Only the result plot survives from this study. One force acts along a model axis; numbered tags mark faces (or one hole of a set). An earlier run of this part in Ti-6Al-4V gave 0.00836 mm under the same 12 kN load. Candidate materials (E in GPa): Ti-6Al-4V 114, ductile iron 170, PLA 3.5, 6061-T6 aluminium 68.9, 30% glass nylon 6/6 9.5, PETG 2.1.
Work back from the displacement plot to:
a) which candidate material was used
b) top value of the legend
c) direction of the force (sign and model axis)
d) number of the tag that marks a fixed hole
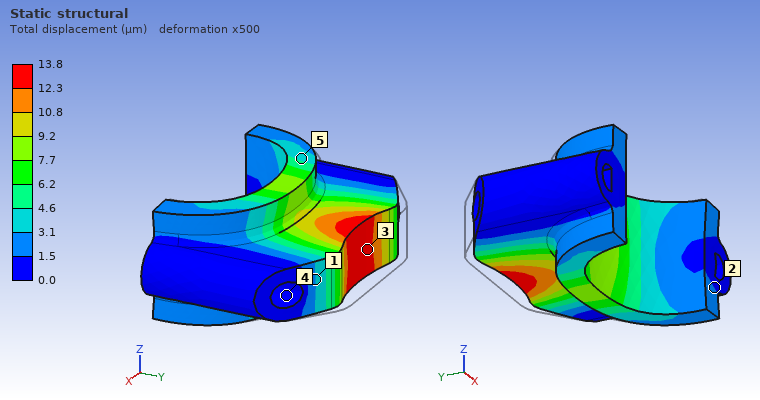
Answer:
6061-T6 aluminium
13.8 µm
-Y
4
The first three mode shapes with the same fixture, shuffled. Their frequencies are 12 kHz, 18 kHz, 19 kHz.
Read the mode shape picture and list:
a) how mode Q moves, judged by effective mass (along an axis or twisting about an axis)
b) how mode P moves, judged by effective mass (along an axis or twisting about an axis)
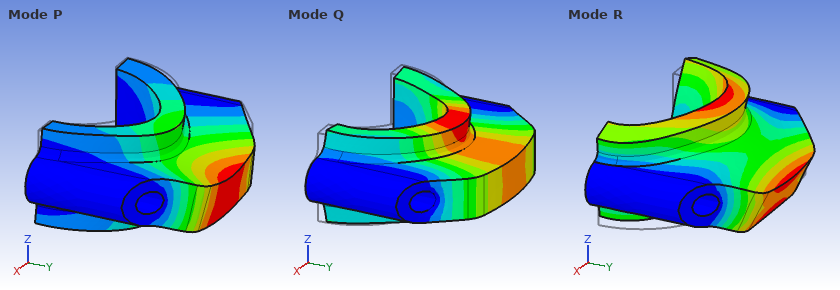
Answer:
along Y
along Z
